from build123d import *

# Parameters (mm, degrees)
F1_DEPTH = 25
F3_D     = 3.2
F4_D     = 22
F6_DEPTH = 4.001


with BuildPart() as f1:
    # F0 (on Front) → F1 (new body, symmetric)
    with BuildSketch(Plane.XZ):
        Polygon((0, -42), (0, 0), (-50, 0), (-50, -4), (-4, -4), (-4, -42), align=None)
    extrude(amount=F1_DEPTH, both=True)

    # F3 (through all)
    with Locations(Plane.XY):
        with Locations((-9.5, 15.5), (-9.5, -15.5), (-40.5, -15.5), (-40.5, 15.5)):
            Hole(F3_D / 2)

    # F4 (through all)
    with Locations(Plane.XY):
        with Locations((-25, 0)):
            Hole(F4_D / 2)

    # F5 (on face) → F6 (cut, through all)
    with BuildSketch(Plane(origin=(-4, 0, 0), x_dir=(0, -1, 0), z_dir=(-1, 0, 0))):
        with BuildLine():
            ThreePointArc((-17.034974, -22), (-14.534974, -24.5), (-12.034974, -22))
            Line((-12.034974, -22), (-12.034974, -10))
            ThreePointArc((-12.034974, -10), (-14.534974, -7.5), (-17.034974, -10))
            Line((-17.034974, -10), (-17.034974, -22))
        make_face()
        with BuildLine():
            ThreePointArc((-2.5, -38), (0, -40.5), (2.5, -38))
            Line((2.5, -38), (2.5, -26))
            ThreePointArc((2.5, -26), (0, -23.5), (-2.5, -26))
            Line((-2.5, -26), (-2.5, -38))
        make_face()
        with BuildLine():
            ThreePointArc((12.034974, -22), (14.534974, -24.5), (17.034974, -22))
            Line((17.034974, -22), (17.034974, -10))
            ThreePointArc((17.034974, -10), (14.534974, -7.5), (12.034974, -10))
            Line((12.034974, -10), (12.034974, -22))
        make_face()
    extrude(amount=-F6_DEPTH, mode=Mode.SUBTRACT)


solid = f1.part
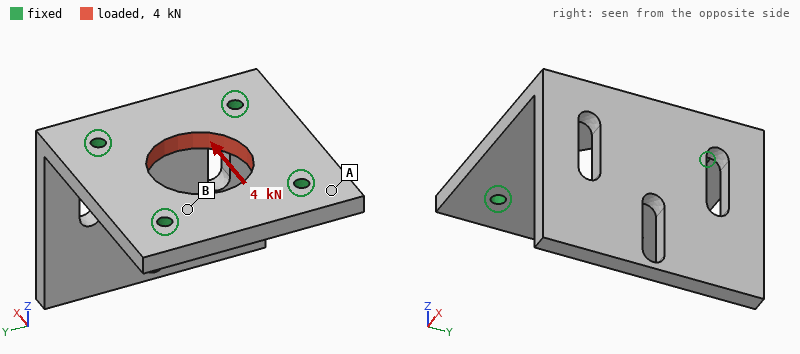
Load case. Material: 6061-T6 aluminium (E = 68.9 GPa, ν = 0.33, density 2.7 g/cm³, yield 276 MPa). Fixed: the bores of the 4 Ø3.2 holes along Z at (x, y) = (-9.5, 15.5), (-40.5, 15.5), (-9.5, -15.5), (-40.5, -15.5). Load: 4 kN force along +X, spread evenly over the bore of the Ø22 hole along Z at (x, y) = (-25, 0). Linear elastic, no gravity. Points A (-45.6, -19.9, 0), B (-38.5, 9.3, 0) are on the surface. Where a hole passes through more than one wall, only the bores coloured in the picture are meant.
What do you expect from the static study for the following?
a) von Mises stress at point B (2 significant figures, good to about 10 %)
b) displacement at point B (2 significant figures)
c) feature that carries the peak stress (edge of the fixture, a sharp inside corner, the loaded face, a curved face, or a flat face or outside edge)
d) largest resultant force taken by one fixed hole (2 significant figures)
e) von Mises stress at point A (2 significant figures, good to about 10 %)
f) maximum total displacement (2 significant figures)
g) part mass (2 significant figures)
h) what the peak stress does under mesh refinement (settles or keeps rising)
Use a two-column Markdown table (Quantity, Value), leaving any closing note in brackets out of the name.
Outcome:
| Quantity | Value |
|---|---|
| von Mises stress at point B | 17 MPa |
| displacement at point B | 3.5 µm |
| feature that carries the peak stress | edge of the fixture |
| largest resultant force taken by one fixed hole | 1.0 kN |
| von Mises stress at point A | 6.2 MPa |
| maximum total displacement | 7.1 µm |
| part mass | 40 g |
| what the peak stress does under mesh refinement | keeps rising |
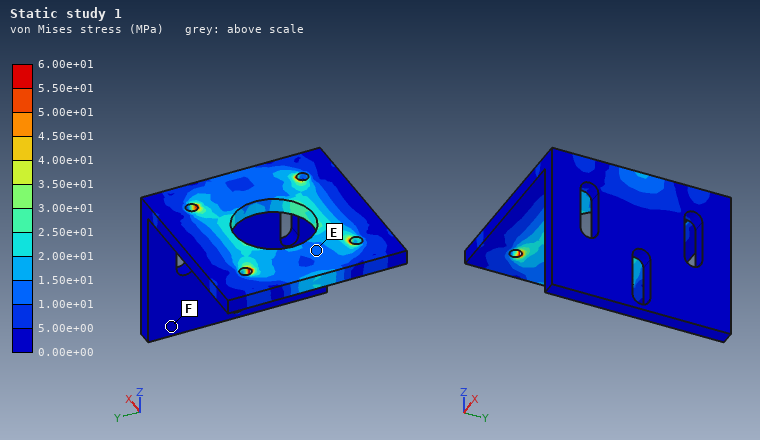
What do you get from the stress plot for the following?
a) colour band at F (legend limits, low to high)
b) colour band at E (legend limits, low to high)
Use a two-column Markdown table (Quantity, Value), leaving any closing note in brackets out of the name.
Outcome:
| Quantity | Value |
|---|---|
| colour band at F | 0.00e+00 to 5.00e+00 MPa |
| colour band at E | 1.00e+01 to 1.50e+01 MPa |
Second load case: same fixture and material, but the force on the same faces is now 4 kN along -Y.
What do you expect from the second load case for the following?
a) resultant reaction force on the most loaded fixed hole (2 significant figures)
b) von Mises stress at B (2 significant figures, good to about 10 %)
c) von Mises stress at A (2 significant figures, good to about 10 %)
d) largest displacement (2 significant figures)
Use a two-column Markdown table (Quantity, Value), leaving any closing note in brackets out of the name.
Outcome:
| Quantity | Value |
|---|---|
| resultant reaction force on the most loaded fixed hole | 1.0 kN |
| von Mises stress at B | 20 MPa |
| von Mises stress at A | 5.9 MPa |
| largest displacement | 6.9 µm |
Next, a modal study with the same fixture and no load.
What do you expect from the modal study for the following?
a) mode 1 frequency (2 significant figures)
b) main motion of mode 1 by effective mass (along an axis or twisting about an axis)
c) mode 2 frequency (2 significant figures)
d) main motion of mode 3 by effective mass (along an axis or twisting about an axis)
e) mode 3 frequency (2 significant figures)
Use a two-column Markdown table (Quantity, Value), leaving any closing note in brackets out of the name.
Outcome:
| Quantity | Value |
|---|---|
| mode 1 frequency | 1600 Hz |
| main motion of mode 1 by effective mass | along X |
| mode 2 frequency | 3300 Hz |
| main motion of mode 3 by effective mass | along Y |
| mode 3 frequency | 6200 Hz |
